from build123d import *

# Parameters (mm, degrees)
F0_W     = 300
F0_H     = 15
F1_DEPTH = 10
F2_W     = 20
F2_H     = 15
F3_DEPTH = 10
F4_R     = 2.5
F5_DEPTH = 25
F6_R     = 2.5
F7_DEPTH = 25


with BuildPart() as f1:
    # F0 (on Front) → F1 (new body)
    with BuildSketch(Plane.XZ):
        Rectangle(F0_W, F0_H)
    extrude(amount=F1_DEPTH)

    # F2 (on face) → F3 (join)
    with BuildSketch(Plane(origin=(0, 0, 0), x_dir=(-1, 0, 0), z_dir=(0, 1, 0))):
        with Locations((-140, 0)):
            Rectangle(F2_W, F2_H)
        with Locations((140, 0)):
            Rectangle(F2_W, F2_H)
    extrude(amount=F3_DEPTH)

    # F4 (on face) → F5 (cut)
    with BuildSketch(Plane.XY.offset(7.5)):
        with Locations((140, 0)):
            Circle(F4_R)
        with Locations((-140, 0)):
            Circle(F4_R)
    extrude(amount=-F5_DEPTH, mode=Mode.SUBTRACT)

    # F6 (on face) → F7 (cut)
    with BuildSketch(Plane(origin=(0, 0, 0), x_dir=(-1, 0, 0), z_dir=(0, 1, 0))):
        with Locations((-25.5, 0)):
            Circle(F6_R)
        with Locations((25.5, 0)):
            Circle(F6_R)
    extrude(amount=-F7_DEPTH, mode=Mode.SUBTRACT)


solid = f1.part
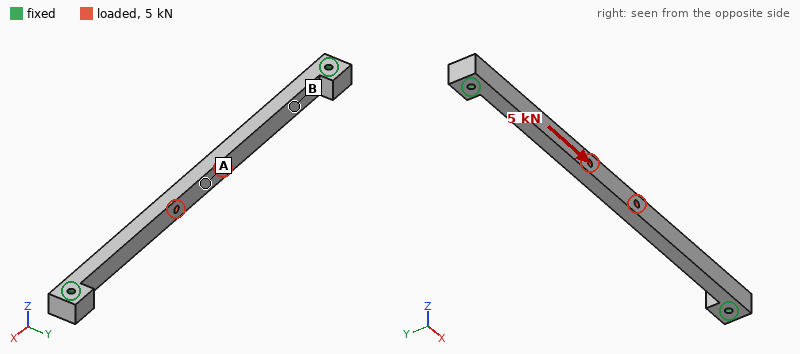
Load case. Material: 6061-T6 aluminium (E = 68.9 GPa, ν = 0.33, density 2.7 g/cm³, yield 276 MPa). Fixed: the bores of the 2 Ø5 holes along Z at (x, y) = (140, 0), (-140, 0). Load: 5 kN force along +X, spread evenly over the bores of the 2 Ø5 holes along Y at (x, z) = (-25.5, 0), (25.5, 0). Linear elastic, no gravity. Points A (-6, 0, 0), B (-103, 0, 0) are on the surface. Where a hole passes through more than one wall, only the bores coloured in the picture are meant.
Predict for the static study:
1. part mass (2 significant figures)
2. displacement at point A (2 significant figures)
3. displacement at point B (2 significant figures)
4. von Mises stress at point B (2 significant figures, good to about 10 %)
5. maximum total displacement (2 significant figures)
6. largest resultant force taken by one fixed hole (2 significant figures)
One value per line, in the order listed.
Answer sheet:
140 g
31 µm
16 µm
20 MPa
33 µm
2.5 kN
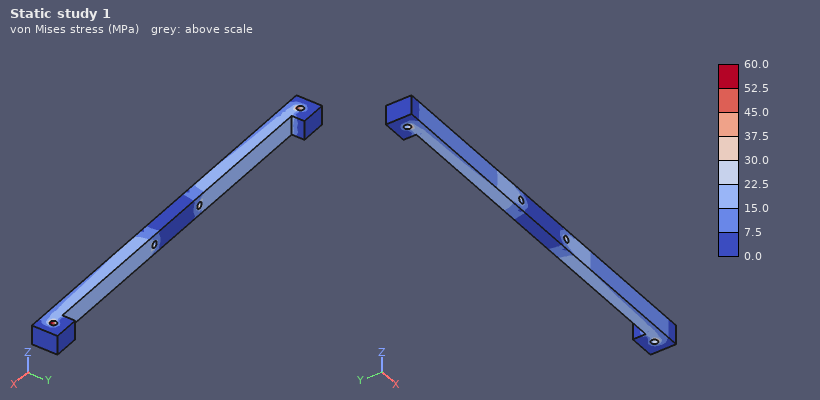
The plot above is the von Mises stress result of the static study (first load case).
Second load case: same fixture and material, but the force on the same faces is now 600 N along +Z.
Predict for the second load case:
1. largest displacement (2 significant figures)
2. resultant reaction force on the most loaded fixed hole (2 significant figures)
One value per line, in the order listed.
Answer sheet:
0.33 mm
300 N
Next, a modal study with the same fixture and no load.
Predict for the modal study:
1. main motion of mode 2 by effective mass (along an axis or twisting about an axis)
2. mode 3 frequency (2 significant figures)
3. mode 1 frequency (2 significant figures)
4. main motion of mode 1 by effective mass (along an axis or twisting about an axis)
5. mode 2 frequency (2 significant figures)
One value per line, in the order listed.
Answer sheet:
along Z
1800 Hz
680 Hz
along Y
1000 Hz
